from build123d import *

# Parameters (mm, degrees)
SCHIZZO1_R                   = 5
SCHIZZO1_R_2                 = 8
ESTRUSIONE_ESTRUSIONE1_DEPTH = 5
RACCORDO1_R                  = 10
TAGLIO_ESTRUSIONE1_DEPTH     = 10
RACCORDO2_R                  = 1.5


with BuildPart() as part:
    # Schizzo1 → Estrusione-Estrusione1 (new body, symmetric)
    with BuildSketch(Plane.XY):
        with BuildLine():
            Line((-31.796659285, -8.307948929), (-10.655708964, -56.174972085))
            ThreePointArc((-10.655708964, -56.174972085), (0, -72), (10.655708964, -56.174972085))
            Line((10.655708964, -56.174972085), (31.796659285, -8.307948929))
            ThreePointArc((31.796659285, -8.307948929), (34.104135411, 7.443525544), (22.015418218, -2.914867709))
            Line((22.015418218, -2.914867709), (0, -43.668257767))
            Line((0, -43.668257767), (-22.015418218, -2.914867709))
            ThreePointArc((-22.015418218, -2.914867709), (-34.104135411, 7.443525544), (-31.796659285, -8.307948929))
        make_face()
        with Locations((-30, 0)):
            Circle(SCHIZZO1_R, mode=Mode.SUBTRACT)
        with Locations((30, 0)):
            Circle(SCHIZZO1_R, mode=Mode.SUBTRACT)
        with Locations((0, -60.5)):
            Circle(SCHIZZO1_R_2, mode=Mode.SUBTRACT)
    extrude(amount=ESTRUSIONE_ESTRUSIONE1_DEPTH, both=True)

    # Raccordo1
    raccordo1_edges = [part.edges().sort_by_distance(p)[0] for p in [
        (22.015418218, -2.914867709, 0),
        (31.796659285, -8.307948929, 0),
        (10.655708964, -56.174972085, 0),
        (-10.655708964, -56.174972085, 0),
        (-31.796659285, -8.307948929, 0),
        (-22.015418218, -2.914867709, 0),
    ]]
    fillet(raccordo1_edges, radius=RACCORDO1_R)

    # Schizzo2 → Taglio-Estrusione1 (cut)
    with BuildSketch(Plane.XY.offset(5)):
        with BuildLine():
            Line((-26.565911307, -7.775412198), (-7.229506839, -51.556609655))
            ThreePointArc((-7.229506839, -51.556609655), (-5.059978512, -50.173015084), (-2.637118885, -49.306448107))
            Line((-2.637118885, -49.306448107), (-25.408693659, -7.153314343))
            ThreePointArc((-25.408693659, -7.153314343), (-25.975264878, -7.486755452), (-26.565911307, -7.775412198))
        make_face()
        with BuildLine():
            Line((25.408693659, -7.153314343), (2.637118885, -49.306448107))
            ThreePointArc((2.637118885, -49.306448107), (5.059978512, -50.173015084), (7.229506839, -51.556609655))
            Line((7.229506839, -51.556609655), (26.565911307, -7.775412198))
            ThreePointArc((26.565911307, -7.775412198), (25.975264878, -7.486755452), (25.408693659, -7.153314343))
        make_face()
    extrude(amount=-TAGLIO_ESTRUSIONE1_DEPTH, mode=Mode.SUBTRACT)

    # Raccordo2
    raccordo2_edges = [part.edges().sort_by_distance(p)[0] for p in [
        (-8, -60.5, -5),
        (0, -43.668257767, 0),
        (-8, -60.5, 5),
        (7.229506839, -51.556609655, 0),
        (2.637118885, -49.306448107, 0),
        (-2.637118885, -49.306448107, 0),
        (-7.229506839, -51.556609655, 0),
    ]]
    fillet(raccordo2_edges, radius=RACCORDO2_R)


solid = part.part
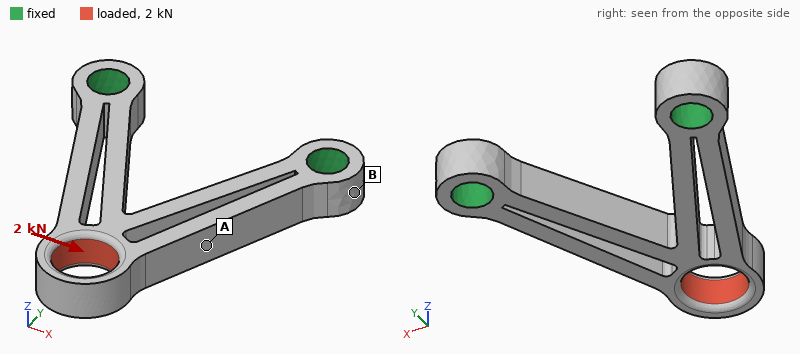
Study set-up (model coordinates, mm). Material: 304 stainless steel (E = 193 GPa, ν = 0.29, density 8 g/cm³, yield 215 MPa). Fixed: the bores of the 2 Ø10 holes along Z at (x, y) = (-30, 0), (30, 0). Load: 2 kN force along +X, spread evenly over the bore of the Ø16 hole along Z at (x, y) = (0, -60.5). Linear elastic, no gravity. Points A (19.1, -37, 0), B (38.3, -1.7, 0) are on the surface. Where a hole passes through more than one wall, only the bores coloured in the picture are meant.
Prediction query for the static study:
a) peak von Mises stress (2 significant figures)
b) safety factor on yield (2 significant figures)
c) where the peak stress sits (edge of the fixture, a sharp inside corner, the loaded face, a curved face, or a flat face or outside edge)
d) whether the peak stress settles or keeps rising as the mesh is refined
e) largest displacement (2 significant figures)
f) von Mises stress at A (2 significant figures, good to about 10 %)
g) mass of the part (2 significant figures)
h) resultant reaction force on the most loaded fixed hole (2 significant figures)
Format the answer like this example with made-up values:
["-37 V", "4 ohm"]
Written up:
["110 MPa", "1.9", "the loaded face", "settles", "36 µm", "33 MPa", "120 g", "2.2 kN"]
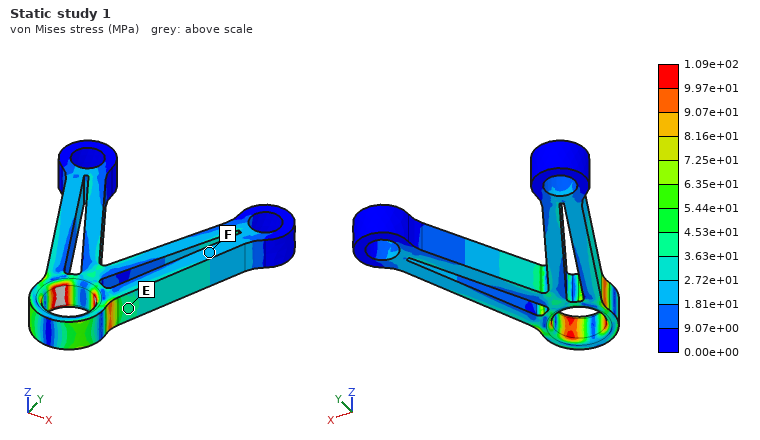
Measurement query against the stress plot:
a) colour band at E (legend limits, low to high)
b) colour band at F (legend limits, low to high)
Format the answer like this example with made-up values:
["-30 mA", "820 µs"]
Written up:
["3.63e+01 to 4.53e+01 MPa", "1.81e+01 to 2.72e+01 MPa"]
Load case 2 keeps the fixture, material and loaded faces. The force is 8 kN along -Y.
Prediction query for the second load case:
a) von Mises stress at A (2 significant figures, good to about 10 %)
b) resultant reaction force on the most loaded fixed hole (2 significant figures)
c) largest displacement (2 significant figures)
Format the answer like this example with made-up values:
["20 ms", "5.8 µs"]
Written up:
["70 MPa", "4.4 kN", "31 µm"]
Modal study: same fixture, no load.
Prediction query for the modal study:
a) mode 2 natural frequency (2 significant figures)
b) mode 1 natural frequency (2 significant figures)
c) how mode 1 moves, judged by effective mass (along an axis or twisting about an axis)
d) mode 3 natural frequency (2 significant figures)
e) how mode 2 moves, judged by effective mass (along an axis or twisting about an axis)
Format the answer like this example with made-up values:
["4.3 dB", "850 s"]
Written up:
["6400 Hz", "1900 Hz", "along Z", "6800 Hz", "along X"]
